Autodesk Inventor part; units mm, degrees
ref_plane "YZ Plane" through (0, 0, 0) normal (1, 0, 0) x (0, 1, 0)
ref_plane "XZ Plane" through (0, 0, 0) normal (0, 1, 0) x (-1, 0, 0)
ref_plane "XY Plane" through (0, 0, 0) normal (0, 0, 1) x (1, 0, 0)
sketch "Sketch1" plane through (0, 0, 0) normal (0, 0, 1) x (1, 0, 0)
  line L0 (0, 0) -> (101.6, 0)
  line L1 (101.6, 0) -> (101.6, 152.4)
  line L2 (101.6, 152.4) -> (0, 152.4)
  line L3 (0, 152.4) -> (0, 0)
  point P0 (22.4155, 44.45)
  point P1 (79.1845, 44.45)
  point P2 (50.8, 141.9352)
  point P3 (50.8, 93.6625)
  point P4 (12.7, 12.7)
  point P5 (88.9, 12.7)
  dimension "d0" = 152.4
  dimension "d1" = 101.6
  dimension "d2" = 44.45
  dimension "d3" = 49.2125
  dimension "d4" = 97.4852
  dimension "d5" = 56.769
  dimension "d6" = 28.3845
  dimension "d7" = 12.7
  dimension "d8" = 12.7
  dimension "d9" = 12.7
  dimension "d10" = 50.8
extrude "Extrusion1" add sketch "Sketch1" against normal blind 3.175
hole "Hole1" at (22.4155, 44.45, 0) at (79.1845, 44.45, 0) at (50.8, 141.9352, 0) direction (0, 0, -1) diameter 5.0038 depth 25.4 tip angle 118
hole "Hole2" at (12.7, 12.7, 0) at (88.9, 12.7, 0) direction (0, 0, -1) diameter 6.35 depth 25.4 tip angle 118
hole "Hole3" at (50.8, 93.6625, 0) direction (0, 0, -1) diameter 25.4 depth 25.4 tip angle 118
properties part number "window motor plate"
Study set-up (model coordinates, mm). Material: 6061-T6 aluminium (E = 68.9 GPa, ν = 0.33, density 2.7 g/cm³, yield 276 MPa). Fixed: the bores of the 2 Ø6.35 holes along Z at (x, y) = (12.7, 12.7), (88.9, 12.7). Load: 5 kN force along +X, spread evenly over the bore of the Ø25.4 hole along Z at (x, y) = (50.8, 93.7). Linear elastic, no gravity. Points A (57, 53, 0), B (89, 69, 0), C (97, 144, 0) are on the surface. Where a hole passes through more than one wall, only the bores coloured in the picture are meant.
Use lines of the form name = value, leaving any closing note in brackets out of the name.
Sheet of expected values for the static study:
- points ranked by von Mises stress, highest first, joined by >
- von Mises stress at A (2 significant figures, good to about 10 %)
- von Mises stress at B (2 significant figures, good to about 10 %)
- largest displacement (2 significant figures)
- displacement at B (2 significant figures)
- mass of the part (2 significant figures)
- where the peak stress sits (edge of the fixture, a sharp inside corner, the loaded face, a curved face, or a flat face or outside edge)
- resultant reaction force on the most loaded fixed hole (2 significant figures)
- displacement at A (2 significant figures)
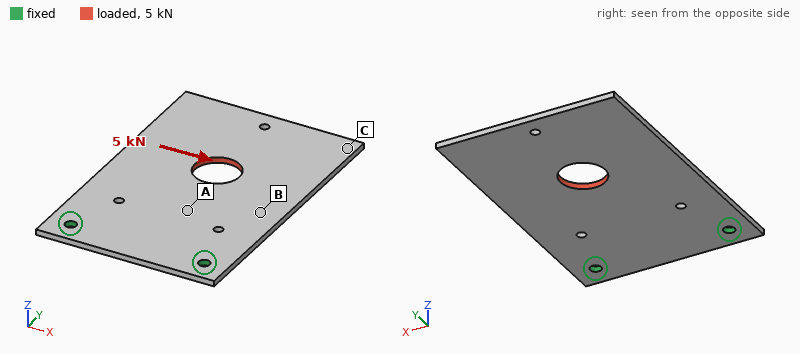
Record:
points ranked by von Mises stress, highest first, joined by > = A > B > C
von Mises stress at A = 43 MPa
von Mises stress at B = 26 MPa
largest displacement = 0.20 mm
displacement at B = 0.086 mm
mass of the part = 130 g
where the peak stress sits = edge of the fixture
resultant reaction force on the most loaded fixed hole = 5.7 kN
displacement at A = 0.052 mm
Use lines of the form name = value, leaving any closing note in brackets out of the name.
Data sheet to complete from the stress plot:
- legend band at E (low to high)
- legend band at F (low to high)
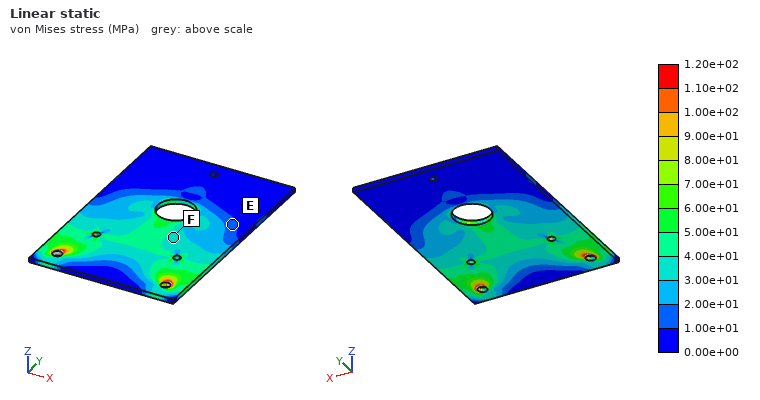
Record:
legend band at E = 1.00e+01 to 2.00e+01 MPa
legend band at F = 3.00e+01 to 4.00e+01 MPa
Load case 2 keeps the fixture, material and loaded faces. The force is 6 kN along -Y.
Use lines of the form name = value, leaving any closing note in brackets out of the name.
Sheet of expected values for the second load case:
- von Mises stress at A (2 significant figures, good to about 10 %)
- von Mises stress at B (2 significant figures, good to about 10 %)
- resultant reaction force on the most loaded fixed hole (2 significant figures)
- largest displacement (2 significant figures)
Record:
von Mises stress at A = 18 MPa
von Mises stress at B = 17 MPa
resultant reaction force on the most loaded fixed hole = 3.1 kN
largest displacement = 42 µm
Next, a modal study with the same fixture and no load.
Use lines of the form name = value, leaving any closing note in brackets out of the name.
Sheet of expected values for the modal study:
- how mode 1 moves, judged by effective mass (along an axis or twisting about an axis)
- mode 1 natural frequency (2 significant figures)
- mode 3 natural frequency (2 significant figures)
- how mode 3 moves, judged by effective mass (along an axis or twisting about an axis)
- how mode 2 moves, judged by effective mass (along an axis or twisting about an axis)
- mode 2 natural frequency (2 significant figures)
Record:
how mode 1 moves, judged by effective mass = along Z
mode 1 natural frequency = 130 Hz
mode 3 natural frequency = 780 Hz
how mode 3 moves, judged by effective mass = along Z
how mode 2 moves, judged by effective mass = twisting about Y
mode 2 natural frequency = 410 Hz
